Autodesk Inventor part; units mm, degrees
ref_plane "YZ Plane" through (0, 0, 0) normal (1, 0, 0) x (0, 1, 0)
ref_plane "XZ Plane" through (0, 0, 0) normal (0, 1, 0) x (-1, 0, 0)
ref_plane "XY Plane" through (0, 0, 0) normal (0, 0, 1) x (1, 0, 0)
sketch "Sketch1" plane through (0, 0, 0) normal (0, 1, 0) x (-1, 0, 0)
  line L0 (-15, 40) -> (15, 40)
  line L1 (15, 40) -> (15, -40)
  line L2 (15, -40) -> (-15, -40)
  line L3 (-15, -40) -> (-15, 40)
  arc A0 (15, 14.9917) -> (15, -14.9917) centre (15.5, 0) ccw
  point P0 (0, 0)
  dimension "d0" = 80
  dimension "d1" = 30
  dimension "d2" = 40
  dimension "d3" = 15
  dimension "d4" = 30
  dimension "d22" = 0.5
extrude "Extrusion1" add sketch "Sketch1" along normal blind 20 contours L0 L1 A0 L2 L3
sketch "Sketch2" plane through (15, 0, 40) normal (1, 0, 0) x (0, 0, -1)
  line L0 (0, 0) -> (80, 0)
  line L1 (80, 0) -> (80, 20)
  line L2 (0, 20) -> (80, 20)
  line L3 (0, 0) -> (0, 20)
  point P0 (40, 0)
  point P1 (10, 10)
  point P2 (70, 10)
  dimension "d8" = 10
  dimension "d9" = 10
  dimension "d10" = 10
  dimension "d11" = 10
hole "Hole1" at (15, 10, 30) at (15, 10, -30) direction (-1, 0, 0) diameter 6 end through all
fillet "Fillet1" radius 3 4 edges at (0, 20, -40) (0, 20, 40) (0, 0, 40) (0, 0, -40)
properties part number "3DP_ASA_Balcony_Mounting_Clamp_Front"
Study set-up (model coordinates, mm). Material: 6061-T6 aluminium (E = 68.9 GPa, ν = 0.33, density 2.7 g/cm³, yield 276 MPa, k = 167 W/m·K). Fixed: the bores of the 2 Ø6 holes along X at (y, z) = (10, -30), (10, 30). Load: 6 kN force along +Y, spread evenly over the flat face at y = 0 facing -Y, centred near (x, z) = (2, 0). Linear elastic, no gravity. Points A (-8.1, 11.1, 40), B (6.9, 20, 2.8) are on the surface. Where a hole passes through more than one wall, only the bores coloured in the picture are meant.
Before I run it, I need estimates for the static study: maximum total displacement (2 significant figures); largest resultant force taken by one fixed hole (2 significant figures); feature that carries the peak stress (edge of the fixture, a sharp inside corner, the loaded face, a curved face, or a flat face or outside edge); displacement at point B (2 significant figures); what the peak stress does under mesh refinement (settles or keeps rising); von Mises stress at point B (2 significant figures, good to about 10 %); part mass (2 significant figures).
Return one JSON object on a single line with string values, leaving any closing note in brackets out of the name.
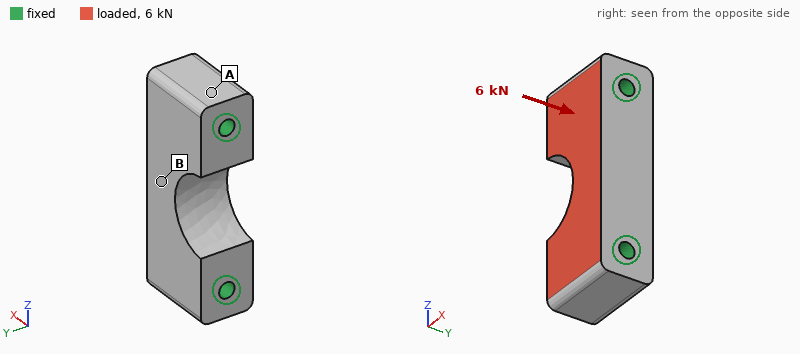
{"maximum total displacement": "7.7 µm", "largest resultant force taken by one fixed hole": "3.0 kN", "feature that carries the peak stress": "edge of the fixture", "displacement at point B": "6.4 µm", "what the peak stress does under mesh refinement": "keeps rising", "von Mises stress at point B": "10 MPa", "part mass": "110 g"}
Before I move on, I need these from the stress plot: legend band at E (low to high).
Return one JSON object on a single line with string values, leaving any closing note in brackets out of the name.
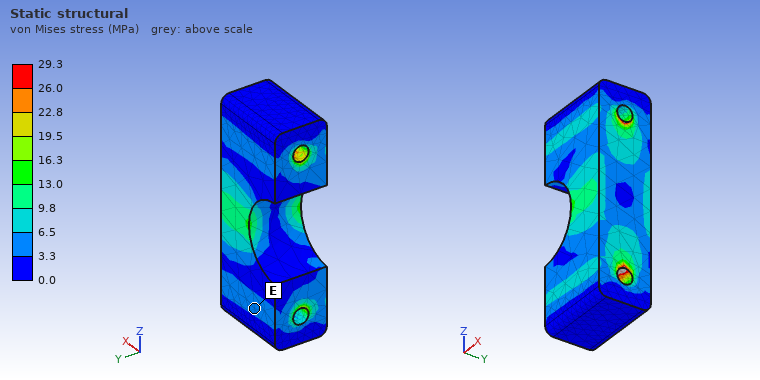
{"legend band at E": "3.3 to 6.5 MPa"}
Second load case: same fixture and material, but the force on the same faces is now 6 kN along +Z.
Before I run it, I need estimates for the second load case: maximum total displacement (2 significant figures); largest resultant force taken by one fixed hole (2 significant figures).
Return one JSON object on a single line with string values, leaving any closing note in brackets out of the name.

{"maximum total displacement": "3.2 µm", "largest resultant force taken by one fixed hole": "3.1 kN"}
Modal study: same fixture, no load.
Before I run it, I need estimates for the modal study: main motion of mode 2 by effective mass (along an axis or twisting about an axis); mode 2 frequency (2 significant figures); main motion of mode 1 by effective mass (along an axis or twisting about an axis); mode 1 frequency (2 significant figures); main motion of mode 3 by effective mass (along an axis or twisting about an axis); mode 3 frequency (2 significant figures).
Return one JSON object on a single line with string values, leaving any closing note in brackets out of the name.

{"main motion of mode 2 by effective mass": "along X", "mode 2 frequency": "24 kHz", "main motion of mode 1 by effective mass": "along Y", "mode 1 frequency": "16 kHz", "main motion of mode 3 by effective mass": "twisting about Z", "mode 3 frequency": "31 kHz"}
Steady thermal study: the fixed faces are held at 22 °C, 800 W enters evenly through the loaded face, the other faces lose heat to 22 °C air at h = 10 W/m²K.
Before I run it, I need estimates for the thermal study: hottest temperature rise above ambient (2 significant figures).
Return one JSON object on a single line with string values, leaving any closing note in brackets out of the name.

{"hottest temperature rise above ambient": "66 K"}
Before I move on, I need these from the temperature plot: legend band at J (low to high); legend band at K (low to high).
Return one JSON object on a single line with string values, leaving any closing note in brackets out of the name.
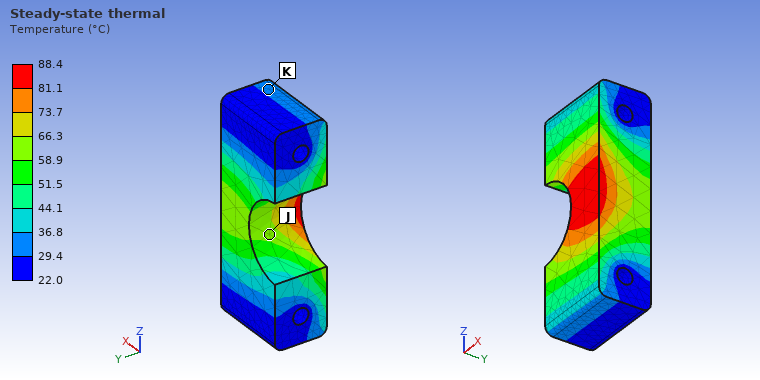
{"legend band at J": "58.9 to 66.3 °C", "legend band at K": "29.4 to 36.8 °C"}
